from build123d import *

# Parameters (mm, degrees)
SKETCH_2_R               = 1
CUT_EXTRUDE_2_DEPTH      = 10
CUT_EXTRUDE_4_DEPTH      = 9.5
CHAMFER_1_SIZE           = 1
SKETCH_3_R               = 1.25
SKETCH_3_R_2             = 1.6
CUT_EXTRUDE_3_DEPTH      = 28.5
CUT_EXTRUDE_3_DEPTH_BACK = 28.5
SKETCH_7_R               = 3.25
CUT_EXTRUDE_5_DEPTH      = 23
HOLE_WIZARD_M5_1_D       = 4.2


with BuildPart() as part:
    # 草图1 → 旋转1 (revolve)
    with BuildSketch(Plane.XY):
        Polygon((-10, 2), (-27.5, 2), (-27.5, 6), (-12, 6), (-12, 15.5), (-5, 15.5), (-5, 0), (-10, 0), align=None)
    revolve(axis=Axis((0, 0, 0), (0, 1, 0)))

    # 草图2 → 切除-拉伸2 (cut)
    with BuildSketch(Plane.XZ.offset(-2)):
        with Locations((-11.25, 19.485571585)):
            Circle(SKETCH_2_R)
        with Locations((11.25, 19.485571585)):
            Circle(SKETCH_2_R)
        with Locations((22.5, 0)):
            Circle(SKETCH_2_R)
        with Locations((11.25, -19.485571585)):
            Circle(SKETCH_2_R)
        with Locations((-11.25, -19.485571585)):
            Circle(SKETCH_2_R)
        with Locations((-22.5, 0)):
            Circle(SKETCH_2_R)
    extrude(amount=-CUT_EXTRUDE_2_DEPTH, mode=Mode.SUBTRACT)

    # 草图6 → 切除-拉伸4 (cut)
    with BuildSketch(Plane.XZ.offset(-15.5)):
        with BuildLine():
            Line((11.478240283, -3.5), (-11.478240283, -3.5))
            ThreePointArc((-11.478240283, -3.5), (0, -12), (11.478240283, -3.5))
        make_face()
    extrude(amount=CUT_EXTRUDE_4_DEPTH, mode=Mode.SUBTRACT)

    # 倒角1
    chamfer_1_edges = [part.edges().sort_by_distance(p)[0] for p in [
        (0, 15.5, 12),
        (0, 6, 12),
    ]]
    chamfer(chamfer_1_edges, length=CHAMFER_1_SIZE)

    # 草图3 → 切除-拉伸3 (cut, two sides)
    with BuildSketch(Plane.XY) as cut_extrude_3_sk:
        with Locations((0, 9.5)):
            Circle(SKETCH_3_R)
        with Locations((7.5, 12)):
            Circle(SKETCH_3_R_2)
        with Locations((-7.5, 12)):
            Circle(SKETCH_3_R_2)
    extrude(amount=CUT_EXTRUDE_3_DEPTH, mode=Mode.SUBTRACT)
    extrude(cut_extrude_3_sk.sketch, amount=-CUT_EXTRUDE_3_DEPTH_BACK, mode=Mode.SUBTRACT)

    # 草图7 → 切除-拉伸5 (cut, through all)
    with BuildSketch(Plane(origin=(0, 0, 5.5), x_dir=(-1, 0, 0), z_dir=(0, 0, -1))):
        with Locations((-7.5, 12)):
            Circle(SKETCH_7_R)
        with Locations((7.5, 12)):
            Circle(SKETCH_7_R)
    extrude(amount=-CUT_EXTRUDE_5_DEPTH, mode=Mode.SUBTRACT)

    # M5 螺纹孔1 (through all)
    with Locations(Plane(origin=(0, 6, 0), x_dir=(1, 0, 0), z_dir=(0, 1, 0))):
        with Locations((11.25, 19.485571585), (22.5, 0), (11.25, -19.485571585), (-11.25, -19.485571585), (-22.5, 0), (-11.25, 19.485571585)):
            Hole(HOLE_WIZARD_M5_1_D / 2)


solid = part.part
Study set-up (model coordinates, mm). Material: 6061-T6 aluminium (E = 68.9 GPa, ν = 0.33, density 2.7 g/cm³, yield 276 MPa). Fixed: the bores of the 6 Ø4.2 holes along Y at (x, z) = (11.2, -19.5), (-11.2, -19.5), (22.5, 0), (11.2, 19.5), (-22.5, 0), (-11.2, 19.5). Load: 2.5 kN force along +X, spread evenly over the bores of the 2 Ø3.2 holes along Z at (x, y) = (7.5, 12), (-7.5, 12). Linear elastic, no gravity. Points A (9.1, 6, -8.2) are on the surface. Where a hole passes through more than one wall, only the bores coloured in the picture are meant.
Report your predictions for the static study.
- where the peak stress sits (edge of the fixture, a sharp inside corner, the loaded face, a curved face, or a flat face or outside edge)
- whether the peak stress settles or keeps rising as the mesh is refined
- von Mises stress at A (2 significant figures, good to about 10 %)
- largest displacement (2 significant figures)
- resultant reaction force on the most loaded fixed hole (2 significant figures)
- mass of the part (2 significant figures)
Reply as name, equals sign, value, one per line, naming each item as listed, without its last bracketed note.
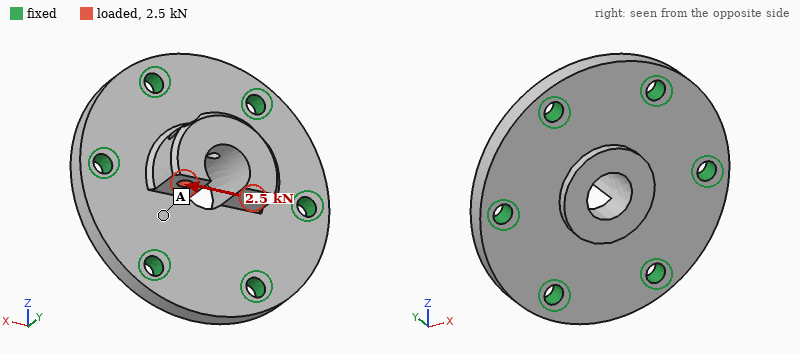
where the peak stress sits = a sharp inside corner
whether the peak stress settles or keeps rising as the mesh is refined = keeps rising
von Mises stress at A = 13 MPa
largest displacement = 27 µm
resultant reaction force on the most loaded fixed hole = 810 N
mass of the part = 30 g
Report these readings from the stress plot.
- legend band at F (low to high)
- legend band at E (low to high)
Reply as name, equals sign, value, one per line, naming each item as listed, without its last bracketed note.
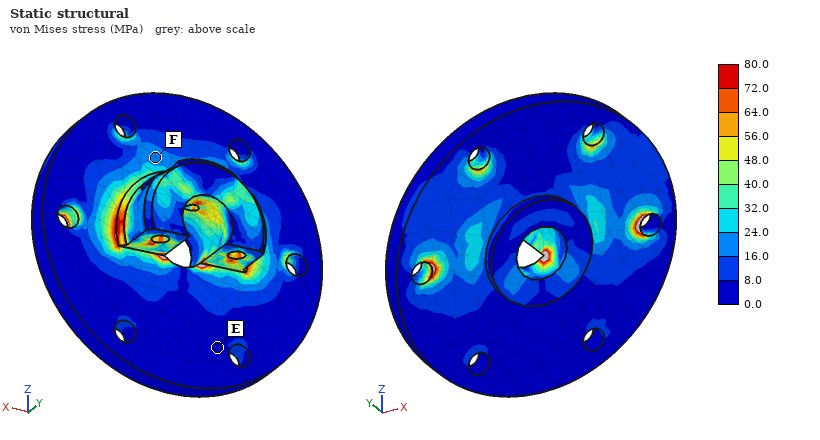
legend band at F = 16.0 to 24.0 MPa
legend band at E = 0.0 to 8.0 MPa
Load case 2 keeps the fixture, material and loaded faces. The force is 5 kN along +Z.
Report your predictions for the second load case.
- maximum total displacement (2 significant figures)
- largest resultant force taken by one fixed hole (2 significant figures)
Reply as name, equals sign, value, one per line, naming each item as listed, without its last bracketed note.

maximum total displacement = 56 µm
largest resultant force taken by one fixed hole = 1.6 kN
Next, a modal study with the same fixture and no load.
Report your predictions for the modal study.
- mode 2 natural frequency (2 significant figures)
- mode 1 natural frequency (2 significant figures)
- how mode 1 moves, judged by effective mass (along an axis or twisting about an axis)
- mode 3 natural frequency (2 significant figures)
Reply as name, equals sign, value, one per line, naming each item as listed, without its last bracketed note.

mode 2 natural frequency = 25 kHz
mode 1 natural frequency = 17 kHz
how mode 1 moves, judged by effective mass = along Y
mode 3 natural frequency = 26 kHz
